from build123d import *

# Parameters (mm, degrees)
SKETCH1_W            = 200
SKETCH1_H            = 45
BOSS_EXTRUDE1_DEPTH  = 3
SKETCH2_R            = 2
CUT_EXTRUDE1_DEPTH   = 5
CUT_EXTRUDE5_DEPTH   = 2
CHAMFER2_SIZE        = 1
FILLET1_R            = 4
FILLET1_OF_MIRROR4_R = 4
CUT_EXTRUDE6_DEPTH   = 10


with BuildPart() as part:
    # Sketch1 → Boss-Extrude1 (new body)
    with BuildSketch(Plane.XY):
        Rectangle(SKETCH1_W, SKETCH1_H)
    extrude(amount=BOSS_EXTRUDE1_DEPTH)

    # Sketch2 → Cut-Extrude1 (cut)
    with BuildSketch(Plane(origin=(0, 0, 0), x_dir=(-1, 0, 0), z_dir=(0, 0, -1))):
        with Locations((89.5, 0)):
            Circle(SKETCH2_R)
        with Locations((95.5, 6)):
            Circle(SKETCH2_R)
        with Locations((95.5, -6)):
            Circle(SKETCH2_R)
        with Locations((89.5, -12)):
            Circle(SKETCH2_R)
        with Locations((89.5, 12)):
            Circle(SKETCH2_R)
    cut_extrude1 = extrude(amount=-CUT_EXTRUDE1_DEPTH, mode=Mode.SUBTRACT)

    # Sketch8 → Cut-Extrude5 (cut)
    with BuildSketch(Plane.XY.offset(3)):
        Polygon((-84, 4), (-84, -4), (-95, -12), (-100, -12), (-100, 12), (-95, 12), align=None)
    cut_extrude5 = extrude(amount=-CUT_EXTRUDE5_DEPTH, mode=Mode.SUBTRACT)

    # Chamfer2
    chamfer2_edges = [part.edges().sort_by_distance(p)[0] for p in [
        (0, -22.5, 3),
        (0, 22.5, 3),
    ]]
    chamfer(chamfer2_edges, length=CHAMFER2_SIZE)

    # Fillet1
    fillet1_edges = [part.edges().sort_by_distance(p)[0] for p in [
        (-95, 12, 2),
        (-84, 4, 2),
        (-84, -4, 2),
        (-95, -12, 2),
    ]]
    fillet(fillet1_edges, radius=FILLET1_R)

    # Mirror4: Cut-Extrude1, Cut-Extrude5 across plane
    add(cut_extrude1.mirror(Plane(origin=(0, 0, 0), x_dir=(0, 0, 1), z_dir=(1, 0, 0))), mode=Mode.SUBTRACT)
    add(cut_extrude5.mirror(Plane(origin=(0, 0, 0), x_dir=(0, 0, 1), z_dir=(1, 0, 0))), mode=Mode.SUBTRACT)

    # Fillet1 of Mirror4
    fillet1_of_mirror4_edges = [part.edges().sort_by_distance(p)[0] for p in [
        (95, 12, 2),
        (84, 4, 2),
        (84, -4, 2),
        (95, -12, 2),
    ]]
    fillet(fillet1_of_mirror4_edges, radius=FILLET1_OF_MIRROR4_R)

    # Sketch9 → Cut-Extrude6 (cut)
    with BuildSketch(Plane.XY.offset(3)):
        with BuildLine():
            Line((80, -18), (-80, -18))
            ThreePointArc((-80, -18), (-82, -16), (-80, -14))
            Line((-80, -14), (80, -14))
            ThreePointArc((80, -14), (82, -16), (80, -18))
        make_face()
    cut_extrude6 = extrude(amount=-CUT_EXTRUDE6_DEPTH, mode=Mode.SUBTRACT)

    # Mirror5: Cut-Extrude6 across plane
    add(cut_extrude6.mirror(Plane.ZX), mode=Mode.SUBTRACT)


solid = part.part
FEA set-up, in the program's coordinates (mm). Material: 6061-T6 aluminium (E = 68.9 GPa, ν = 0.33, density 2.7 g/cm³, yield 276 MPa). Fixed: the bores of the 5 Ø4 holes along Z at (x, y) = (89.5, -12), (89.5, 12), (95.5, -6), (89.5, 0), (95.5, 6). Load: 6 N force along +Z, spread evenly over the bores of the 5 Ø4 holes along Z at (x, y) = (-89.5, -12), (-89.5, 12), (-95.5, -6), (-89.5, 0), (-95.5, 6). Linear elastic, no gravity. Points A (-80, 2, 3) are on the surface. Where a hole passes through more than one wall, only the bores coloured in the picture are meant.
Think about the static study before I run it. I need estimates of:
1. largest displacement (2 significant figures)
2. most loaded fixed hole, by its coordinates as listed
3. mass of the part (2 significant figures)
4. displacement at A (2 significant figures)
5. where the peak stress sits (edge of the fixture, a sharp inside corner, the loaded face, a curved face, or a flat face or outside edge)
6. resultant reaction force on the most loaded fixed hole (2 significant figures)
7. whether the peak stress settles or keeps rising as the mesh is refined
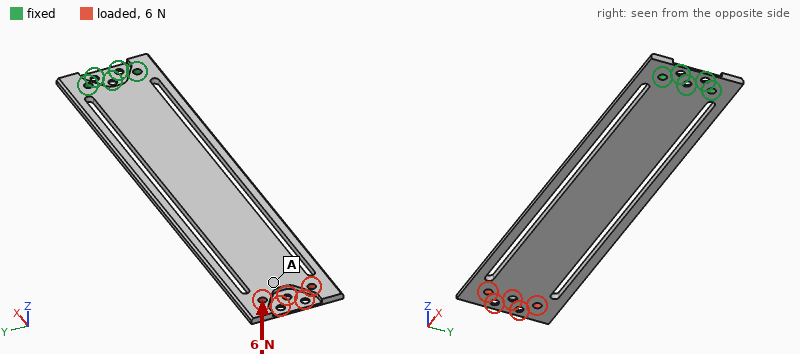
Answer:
2.2 mm
(89.5, 0)
58 g
1.9 mm
edge of the fixture
95 N
keeps rising
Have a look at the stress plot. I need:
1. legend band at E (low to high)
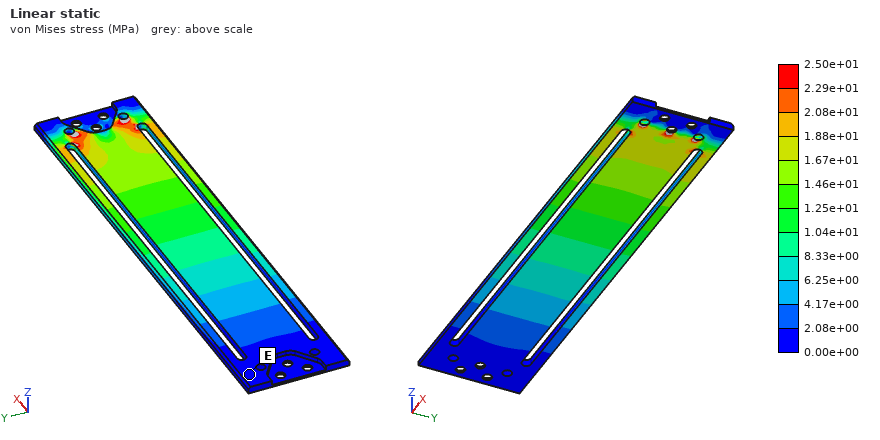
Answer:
0.00e+00 to 2.08e+00 MPa
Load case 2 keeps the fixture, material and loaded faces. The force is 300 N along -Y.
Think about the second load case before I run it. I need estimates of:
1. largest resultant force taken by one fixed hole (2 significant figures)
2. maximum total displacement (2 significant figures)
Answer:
2.0 kN
0.86 mm
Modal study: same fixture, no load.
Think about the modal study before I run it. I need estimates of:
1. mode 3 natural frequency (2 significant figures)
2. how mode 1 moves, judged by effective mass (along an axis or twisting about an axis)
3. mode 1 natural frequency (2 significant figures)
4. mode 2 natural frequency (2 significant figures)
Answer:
440 Hz
along Z
70 Hz
440 Hz
